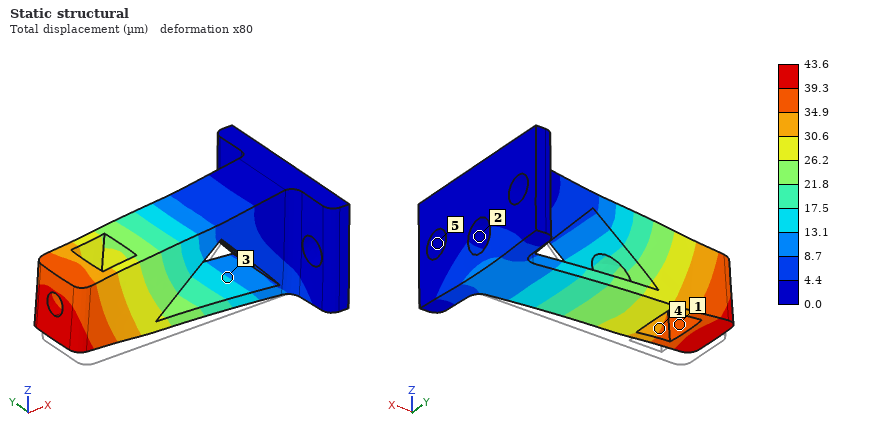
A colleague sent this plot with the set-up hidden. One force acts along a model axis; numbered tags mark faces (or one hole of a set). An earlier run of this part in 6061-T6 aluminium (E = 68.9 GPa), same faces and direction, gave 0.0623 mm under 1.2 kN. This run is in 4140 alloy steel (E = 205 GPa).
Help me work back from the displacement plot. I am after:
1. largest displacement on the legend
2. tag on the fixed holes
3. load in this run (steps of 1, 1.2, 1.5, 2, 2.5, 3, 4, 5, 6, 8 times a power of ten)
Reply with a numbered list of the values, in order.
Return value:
1. 43.6 µm
2. 5
3. 2.5 kN
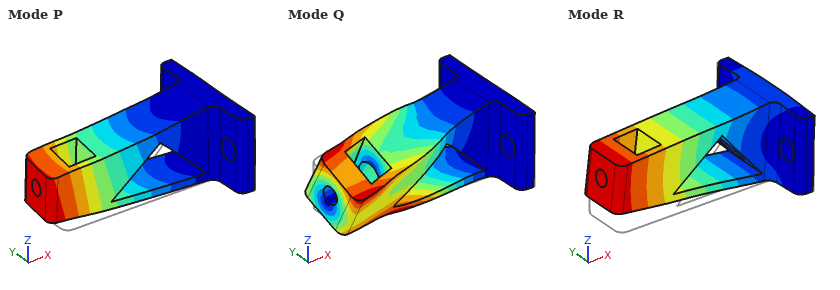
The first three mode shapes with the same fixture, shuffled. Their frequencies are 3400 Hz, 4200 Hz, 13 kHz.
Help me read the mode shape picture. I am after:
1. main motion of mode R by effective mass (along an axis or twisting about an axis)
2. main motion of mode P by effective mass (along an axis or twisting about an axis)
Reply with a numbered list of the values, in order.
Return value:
1. along Z
2. along Y
